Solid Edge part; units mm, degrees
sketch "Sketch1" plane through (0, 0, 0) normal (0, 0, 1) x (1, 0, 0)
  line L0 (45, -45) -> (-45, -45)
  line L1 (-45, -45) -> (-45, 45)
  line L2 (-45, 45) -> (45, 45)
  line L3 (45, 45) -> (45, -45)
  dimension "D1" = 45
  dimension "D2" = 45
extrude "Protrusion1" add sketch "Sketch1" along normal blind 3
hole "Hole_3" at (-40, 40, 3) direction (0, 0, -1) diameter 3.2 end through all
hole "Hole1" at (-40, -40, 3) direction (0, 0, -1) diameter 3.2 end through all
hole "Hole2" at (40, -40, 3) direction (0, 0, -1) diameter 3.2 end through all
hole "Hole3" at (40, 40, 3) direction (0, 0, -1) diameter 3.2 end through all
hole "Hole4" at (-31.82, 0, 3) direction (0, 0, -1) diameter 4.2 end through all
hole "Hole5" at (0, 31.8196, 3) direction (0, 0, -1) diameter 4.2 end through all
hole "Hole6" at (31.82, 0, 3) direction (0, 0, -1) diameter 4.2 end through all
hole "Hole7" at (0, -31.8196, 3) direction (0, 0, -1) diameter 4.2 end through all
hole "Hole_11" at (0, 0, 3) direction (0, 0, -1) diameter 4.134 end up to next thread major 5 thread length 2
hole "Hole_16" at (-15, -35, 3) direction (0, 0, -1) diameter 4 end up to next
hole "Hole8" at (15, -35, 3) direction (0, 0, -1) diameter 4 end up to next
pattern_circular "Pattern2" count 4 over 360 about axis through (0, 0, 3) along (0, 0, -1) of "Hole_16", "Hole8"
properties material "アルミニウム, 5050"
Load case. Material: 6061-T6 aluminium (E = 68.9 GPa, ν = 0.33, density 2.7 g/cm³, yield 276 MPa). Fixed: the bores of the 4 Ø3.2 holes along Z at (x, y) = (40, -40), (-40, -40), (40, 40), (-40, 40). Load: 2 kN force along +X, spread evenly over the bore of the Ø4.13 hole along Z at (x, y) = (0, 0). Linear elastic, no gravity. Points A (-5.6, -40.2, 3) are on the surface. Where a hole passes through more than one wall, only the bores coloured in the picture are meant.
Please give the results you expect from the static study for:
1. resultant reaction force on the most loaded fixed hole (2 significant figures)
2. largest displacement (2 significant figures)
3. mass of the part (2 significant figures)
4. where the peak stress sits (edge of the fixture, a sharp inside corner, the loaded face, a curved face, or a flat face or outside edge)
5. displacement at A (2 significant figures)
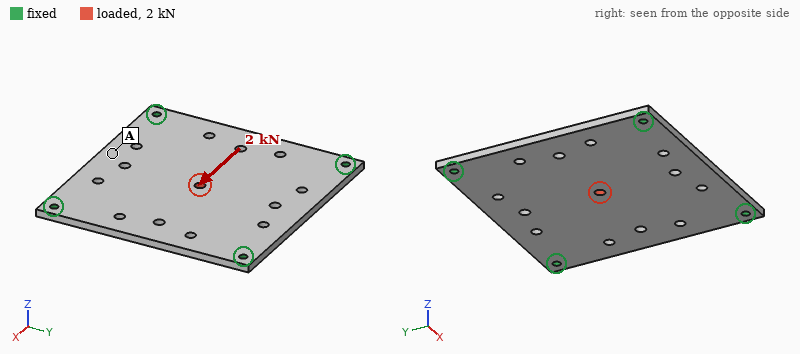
570 N
14 µm
64 g
the loaded face
3.4 µm
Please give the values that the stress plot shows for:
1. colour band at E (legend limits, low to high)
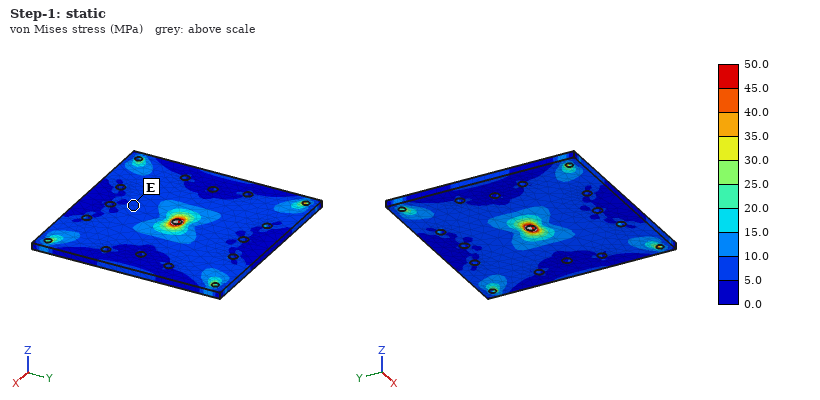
5.0 to 10.0 MPa
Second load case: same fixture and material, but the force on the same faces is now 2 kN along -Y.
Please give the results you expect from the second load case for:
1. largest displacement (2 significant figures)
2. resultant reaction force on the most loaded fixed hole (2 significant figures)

14 µm
570 N
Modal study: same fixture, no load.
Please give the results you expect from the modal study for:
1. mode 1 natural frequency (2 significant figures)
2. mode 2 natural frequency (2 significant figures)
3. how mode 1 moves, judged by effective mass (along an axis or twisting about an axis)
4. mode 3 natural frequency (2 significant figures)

1500 Hz
2600 Hz
along Z
2600 Hz
